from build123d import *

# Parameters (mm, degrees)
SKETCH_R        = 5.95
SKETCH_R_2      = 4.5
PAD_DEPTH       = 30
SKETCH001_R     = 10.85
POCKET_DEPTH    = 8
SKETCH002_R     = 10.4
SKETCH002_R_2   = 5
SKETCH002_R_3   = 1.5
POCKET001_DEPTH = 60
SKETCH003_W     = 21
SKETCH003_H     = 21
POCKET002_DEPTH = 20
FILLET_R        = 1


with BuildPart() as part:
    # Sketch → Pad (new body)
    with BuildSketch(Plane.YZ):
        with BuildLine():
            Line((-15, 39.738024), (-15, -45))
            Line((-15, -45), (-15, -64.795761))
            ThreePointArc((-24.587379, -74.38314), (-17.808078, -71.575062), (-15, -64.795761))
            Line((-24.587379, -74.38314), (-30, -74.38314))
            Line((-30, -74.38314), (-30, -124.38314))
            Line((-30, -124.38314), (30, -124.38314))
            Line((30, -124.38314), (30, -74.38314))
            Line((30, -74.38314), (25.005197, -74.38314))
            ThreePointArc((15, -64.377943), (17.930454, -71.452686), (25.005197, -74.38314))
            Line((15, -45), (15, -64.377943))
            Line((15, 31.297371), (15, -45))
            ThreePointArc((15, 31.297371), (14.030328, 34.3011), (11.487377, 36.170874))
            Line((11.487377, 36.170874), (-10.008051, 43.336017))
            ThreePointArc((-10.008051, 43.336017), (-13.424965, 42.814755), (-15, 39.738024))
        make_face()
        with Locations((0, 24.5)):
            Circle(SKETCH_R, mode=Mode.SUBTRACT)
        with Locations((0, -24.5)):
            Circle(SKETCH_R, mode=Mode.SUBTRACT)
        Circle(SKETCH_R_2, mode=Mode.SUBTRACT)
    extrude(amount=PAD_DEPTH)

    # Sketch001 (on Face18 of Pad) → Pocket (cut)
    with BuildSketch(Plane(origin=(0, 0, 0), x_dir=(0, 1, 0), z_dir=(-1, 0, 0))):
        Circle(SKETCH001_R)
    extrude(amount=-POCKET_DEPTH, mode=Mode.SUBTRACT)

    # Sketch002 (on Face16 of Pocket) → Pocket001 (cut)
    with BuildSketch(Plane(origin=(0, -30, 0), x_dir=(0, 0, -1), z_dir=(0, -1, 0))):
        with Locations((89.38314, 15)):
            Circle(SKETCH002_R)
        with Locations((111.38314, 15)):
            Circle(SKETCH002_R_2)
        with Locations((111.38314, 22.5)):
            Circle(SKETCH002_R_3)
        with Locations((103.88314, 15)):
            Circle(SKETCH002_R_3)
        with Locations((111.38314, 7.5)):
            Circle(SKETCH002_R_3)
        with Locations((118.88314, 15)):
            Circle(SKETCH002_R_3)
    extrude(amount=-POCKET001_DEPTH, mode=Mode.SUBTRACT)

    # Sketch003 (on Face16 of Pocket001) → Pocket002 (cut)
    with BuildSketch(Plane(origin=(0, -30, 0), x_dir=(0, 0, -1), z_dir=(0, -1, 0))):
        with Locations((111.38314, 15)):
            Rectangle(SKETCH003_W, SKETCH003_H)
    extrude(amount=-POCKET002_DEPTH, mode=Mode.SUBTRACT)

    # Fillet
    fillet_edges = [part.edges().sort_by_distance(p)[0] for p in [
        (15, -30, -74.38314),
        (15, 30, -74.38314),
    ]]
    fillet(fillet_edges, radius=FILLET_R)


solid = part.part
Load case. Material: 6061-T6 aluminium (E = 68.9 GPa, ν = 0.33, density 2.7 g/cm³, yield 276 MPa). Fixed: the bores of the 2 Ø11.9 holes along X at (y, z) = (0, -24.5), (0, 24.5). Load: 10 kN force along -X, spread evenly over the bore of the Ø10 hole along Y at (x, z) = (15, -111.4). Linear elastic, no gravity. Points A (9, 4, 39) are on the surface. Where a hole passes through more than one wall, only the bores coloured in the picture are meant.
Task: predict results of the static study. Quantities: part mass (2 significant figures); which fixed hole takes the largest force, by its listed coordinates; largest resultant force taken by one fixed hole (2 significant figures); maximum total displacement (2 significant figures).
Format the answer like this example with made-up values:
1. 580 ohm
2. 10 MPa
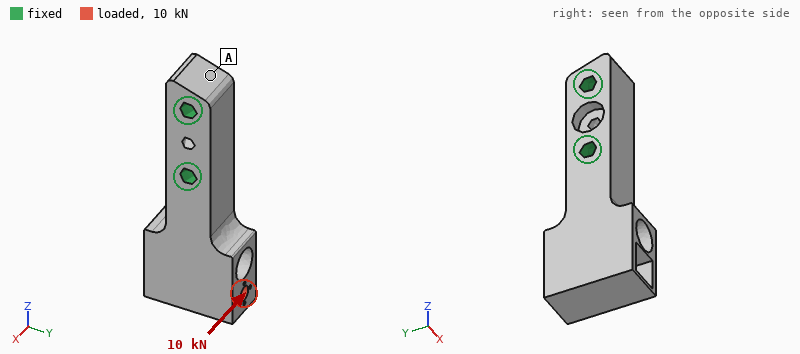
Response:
1. 400 g
2. (0, -24.5)
3. 11 kN
4. 0.71 mm
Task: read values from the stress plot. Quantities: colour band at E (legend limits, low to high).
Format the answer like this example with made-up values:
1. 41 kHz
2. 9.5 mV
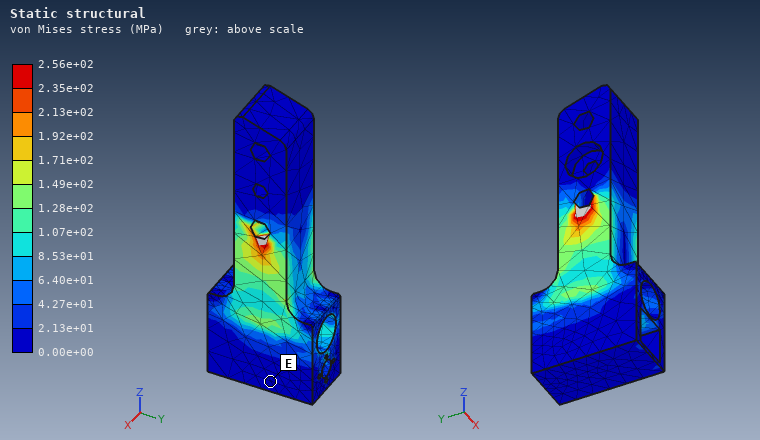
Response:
1. 0.00e+00 to 2.13e+01 MPa
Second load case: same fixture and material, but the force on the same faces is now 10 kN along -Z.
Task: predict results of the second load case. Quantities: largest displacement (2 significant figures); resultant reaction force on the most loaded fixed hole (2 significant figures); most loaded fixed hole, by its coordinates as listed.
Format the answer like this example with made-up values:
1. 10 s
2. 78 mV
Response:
1. 0.13 mm
2. 9.6 kN
3. (0, -24.5)
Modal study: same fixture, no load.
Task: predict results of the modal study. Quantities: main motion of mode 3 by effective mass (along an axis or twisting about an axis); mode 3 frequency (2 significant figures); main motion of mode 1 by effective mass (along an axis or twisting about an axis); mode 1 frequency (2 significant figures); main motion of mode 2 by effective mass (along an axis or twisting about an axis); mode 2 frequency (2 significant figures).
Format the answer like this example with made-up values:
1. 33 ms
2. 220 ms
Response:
1. twisting about Z
2. 4400 Hz
3. along Y
4. 1800 Hz
5. along X
6. 2000 Hz
